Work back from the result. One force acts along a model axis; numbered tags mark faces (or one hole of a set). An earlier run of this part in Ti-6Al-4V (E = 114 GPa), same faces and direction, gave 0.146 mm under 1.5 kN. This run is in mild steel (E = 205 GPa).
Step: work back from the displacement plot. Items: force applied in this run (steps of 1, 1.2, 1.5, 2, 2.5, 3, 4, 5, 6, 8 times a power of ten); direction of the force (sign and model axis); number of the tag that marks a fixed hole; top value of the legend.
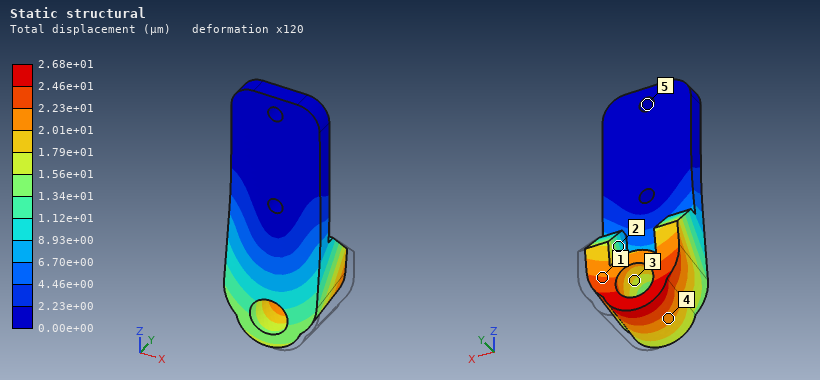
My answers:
500 N
-X
5
2.68e+01 µm
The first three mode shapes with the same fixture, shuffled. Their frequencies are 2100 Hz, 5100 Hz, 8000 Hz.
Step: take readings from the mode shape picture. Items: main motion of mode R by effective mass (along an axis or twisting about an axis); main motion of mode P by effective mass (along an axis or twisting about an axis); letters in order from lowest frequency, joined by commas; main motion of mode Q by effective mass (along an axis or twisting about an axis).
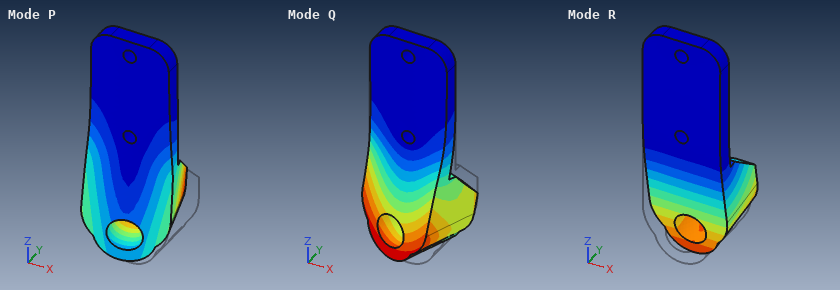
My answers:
along Y
along X
R, P, Q
along X
